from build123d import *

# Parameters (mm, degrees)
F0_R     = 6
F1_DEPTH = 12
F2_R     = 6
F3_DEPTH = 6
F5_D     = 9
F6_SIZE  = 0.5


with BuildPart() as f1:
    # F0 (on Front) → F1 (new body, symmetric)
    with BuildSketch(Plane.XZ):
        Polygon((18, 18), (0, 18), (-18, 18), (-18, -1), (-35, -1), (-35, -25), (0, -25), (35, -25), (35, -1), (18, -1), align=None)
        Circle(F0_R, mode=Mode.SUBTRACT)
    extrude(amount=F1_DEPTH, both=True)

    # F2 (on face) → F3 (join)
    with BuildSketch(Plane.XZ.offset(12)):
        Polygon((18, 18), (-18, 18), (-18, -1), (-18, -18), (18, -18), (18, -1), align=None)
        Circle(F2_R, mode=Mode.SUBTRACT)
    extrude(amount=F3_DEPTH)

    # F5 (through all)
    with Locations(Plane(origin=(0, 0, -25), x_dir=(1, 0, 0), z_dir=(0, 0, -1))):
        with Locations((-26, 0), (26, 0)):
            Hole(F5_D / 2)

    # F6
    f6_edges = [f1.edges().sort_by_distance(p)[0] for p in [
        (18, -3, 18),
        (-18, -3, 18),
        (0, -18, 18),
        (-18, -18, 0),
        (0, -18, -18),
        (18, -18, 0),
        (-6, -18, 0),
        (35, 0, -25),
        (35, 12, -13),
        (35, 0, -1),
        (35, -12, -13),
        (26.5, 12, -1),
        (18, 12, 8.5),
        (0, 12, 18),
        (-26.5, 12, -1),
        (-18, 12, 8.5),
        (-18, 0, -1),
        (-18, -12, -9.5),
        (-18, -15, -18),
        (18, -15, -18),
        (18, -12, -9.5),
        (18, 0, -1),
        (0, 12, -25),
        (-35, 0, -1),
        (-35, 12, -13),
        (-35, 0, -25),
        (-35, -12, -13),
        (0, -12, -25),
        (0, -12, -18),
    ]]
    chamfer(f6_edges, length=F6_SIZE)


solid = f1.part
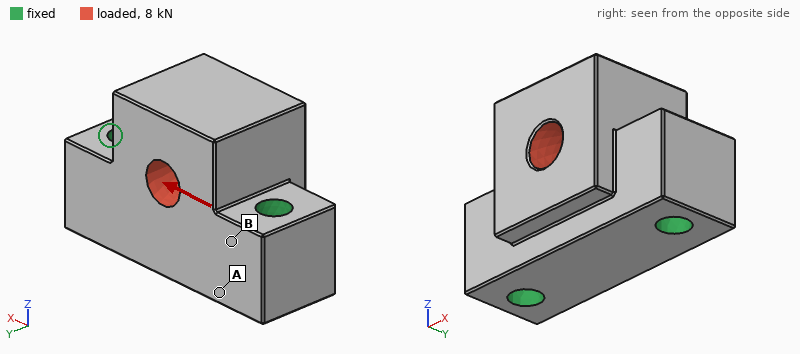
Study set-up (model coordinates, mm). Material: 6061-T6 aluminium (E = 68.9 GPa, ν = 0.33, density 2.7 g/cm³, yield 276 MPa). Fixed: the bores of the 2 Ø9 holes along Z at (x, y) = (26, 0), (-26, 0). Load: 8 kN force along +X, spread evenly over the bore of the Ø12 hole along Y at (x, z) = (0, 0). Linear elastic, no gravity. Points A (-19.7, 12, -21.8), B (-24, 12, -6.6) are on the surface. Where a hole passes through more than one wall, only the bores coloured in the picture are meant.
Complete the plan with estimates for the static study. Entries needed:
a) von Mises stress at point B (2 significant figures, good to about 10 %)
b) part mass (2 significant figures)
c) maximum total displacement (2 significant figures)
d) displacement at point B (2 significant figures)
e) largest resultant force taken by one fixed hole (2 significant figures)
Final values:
6.2 MPa
160 g
6.2 µm
1.2 µm
4.4 kN
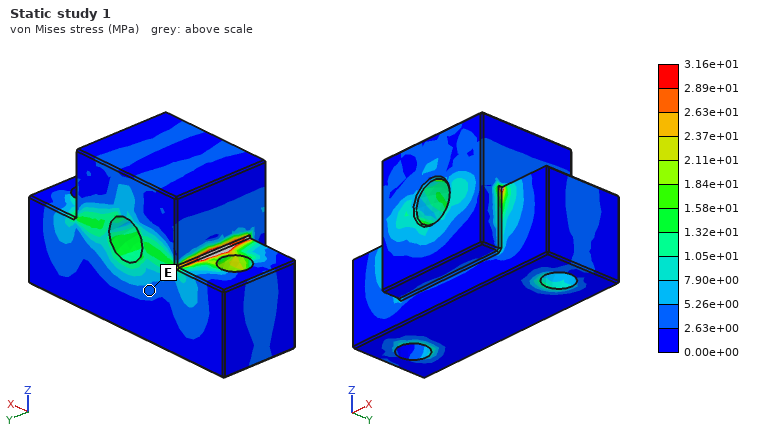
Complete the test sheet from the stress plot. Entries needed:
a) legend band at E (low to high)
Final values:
2.63e+00 to 5.26e+00 MPa
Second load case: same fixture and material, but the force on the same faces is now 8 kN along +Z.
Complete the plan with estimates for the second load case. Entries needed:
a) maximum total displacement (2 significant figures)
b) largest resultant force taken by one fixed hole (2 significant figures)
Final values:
8.5 µm
4.1 kN
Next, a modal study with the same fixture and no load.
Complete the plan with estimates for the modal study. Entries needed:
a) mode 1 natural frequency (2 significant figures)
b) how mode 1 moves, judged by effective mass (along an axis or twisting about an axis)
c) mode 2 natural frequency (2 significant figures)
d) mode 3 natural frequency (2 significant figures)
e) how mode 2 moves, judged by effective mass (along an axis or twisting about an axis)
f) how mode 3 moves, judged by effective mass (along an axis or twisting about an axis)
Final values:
10 kHz
along Y
19 kHz
20 kHz
along X
along Z
